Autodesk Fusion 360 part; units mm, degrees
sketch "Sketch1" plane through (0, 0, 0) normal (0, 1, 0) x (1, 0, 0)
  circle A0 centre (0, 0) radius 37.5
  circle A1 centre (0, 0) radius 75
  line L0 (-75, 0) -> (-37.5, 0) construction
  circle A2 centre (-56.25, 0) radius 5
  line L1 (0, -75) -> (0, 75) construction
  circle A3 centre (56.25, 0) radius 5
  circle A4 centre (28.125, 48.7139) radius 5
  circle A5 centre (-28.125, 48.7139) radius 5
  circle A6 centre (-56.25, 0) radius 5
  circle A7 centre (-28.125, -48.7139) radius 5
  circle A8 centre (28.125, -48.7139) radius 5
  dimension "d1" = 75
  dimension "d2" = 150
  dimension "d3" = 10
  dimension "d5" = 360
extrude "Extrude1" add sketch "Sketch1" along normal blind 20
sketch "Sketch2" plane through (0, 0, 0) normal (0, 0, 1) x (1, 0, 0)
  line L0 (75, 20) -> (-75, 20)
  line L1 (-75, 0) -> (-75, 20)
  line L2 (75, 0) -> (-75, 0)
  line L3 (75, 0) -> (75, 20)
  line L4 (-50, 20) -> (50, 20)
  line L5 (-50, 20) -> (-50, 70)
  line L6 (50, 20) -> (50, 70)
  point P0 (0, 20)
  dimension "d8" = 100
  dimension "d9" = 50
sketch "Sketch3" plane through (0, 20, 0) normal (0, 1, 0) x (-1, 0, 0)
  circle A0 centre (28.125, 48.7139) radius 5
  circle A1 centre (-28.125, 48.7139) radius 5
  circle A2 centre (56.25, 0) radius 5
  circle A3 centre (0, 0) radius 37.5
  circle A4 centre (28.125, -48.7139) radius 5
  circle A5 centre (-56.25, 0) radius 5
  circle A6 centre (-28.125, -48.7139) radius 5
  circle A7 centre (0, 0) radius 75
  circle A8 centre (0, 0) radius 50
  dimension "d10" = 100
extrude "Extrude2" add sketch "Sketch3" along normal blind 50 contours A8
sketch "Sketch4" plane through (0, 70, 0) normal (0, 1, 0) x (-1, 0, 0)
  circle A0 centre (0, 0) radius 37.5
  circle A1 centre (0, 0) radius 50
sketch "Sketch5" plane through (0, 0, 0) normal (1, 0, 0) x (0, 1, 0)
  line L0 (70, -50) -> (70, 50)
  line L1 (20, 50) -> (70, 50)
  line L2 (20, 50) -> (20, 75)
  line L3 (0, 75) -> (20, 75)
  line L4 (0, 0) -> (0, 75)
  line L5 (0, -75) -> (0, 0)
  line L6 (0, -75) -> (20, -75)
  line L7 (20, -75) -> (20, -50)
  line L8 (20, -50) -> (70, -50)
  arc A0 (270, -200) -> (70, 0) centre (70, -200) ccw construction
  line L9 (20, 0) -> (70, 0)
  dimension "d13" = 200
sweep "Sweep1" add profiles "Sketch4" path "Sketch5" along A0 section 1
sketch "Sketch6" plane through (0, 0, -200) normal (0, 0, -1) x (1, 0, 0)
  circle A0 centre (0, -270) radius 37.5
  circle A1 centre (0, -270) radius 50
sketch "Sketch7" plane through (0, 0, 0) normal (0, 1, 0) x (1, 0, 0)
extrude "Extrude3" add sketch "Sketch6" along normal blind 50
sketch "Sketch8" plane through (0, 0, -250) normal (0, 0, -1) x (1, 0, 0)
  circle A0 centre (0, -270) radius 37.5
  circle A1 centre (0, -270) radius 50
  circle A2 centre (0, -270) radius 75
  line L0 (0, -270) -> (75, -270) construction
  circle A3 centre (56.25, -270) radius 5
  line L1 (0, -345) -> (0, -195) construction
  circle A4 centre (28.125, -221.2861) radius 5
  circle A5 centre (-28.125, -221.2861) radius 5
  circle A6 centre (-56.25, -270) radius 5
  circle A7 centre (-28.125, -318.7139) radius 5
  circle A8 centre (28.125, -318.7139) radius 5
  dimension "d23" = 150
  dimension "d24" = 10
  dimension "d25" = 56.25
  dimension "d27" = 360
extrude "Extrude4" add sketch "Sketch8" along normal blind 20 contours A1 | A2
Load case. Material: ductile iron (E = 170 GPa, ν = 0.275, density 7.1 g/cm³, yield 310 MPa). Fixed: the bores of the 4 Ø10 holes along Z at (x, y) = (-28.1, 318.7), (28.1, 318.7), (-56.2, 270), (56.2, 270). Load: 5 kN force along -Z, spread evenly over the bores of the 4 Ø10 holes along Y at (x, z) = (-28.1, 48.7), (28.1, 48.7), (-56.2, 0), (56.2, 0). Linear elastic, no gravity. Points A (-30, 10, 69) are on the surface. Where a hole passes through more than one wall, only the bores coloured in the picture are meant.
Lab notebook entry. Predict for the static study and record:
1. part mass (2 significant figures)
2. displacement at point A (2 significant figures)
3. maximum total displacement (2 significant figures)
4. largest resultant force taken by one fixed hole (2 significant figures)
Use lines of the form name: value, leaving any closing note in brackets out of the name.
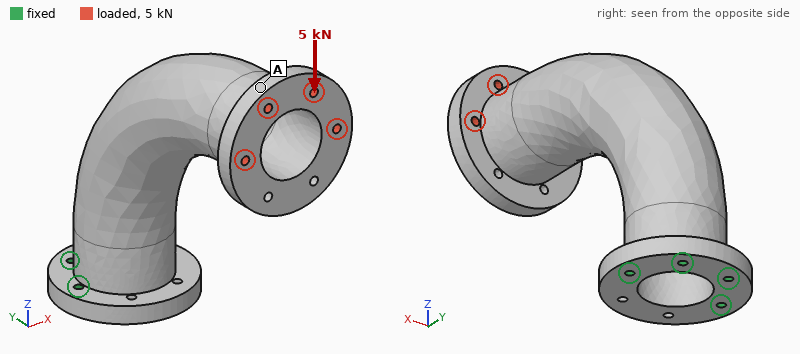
part mass: 14 kg
displacement at point A: 0.37 mm
maximum total displacement: 0.39 mm
largest resultant force taken by one fixed hole: 14 kN
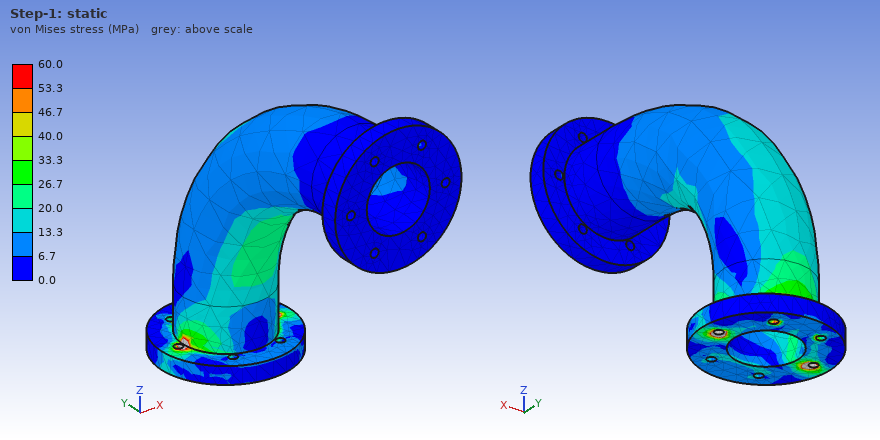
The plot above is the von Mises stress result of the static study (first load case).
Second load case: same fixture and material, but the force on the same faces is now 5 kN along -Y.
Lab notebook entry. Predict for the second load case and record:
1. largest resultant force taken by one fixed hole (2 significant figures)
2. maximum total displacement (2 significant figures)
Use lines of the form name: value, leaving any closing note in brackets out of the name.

largest resultant force taken by one fixed hole: 13 kN
maximum total displacement: 0.31 mm
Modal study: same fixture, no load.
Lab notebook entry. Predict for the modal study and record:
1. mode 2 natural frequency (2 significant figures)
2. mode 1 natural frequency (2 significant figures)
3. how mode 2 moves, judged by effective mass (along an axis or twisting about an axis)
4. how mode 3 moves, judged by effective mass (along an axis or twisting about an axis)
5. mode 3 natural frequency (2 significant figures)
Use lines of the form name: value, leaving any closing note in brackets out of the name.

mode 2 natural frequency: 330 Hz
mode 1 natural frequency: 250 Hz
how mode 2 moves, judged by effective mass: along X
how mode 3 moves, judged by effective mass: along Y
mode 3 natural frequency: 1000 Hz
